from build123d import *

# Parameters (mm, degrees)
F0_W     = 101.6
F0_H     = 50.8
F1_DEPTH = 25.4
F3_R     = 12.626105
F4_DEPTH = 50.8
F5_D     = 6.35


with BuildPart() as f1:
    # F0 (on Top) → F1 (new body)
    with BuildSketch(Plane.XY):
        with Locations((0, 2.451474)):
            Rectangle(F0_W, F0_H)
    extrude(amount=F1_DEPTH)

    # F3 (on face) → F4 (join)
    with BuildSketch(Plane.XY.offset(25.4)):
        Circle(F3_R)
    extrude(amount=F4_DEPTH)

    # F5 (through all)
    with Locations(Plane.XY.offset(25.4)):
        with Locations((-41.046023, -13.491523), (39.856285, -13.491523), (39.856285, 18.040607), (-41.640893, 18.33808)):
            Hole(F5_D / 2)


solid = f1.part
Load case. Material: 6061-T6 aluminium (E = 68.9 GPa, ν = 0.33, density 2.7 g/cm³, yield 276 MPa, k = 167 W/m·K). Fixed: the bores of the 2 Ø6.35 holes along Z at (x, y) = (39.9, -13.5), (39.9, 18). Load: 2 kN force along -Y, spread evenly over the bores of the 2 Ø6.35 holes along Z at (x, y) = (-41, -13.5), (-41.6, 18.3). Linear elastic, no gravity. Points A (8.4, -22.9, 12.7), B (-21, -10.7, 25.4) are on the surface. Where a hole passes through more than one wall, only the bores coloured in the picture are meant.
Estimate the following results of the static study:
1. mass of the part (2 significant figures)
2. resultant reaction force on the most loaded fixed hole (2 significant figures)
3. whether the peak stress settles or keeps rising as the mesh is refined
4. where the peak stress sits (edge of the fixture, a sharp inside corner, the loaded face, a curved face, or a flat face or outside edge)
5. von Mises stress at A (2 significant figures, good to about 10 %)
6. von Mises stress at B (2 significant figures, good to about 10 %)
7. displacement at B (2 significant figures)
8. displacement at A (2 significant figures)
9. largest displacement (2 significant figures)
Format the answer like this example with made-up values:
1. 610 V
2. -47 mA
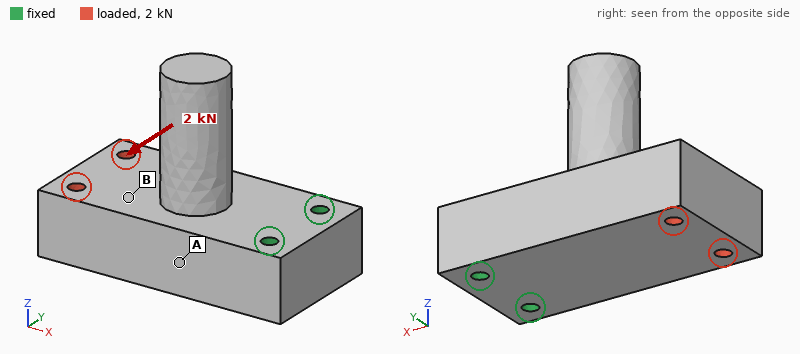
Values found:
1. 410 g
2. 4.8 kN
3. keeps rising
4. edge of the fixture
5. 8.9 MPa
6. 3.6 MPa
7. 17 µm
8. 9.1 µm
9. 31 µm
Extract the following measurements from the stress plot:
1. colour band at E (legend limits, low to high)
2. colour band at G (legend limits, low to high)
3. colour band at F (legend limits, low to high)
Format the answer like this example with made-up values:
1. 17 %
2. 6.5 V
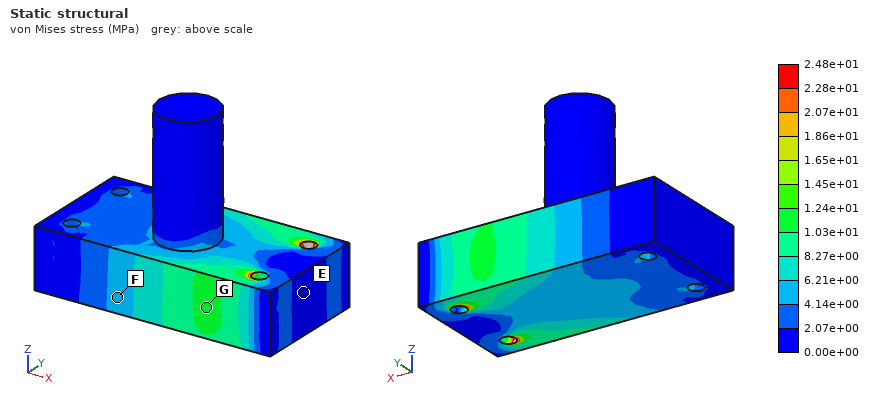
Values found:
1. 0.00e+00 to 2.07e+00 MPa
2. 1.03e+01 to 1.24e+01 MPa
3. 4.14e+00 to 6.21e+00 MPa
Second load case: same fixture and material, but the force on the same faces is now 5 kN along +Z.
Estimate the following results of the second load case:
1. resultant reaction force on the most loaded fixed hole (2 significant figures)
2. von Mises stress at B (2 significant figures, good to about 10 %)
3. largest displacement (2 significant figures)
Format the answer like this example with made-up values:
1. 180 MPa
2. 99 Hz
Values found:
1. 2.5 kN
2. 19 MPa
3. 0.25 mm
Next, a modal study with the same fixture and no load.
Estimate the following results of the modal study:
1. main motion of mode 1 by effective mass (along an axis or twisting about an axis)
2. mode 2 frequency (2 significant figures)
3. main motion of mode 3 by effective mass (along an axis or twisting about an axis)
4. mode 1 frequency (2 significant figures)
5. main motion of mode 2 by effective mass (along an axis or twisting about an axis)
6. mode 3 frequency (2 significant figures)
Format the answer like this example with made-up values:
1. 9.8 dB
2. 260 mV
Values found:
1. along Z
2. 3500 Hz
3. along Y
4. 2100 Hz
5. along Y
6. 4300 Hz
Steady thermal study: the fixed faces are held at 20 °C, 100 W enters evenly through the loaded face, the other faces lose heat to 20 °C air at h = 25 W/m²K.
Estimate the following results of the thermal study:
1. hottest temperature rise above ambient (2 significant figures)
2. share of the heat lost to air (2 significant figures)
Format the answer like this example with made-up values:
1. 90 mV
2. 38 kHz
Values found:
1. 38 K
2. 9.4 %
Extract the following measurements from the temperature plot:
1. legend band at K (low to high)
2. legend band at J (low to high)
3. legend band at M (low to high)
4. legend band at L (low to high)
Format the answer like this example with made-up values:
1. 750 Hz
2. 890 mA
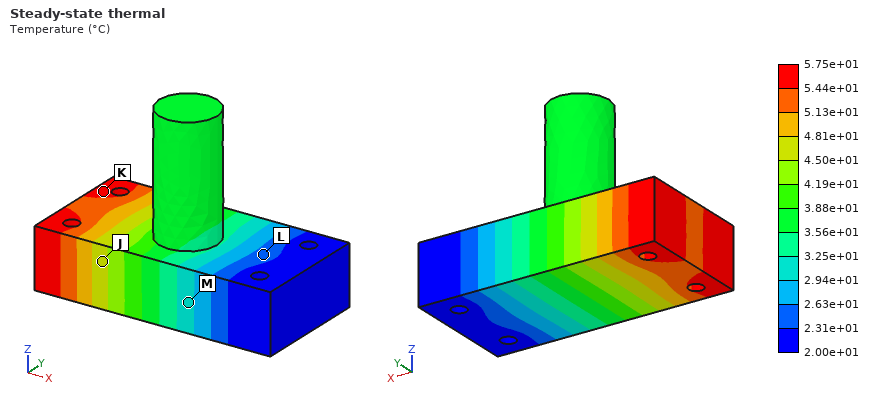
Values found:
1. 5.44e+01 to 5.75e+01 °C
2. 4.50e+01 to 4.81e+01 °C
3. 2.94e+01 to 3.25e+01 °C
4. 2.31e+01 to 2.63e+01 °C
